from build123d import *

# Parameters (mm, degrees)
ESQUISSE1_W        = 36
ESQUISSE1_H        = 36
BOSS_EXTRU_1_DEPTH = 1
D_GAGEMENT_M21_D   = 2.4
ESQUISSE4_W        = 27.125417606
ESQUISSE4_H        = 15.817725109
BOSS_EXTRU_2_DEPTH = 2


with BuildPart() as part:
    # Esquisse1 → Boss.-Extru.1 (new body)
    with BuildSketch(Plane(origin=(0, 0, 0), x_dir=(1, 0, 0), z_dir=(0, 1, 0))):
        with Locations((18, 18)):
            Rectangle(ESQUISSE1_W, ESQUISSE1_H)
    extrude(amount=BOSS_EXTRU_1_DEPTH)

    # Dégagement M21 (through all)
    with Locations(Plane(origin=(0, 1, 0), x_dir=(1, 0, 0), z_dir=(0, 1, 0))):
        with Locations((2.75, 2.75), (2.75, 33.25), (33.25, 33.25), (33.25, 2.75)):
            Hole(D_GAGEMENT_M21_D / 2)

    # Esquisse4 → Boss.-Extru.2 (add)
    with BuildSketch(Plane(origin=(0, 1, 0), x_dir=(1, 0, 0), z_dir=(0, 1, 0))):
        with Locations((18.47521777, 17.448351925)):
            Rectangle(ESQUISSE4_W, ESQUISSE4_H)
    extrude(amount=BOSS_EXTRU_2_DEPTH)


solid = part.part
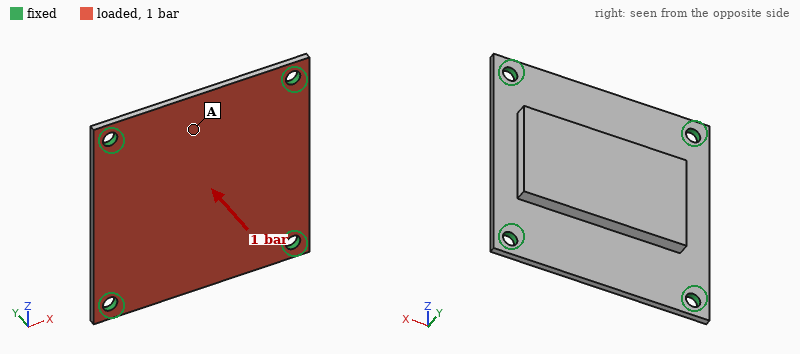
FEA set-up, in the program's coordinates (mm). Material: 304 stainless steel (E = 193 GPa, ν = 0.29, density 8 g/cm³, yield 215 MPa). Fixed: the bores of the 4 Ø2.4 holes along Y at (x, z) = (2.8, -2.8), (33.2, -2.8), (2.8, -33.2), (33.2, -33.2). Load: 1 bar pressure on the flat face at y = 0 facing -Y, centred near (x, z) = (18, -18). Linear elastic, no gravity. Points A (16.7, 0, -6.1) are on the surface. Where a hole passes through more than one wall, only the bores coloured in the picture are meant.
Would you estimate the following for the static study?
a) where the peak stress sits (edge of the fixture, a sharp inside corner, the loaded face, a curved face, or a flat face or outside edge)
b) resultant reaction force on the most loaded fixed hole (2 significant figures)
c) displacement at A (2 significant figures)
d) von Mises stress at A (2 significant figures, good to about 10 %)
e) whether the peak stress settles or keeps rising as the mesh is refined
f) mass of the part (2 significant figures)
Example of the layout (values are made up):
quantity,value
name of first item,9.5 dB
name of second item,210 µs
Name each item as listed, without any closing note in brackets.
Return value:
quantity,value
where the peak stress sits,edge of the fixture
resultant reaction force on the most loaded fixed hole,39 N
displacement at A,8.7 µm
von Mises stress at A,9.0 MPa
whether the peak stress settles or keeps rising as the mesh is refined,keeps rising
mass of the part,17 g
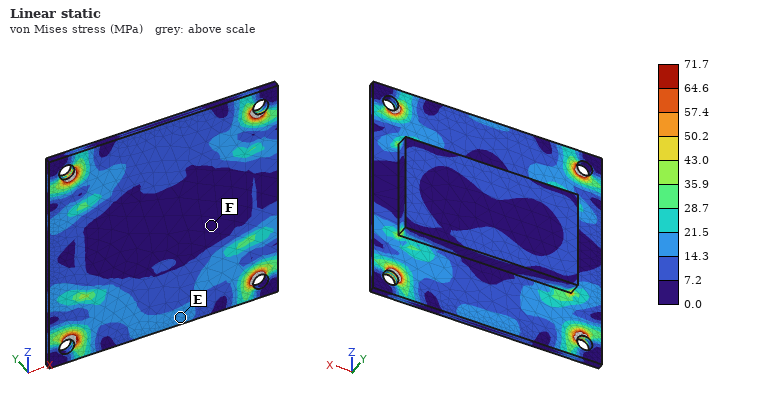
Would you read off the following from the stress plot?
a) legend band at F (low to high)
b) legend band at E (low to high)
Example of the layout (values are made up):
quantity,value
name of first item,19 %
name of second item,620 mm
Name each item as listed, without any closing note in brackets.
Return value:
quantity,value
legend band at F,0.0 to 7.2 MPa
legend band at E,14.3 to 21.5 MPa
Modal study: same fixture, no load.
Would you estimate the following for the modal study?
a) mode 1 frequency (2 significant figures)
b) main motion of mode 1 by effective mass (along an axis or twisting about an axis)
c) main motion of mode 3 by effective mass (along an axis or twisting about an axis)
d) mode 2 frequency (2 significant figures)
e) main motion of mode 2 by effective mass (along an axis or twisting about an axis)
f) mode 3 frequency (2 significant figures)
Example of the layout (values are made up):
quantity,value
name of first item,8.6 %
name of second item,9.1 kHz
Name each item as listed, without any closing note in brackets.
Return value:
quantity,value
mode 1 frequency,4500 Hz
main motion of mode 1 by effective mass,along Y
main motion of mode 3 by effective mass,twisting about X
mode 2 frequency,7400 Hz
main motion of mode 2 by effective mass,twisting about Z
mode 3 frequency,7900 Hz
